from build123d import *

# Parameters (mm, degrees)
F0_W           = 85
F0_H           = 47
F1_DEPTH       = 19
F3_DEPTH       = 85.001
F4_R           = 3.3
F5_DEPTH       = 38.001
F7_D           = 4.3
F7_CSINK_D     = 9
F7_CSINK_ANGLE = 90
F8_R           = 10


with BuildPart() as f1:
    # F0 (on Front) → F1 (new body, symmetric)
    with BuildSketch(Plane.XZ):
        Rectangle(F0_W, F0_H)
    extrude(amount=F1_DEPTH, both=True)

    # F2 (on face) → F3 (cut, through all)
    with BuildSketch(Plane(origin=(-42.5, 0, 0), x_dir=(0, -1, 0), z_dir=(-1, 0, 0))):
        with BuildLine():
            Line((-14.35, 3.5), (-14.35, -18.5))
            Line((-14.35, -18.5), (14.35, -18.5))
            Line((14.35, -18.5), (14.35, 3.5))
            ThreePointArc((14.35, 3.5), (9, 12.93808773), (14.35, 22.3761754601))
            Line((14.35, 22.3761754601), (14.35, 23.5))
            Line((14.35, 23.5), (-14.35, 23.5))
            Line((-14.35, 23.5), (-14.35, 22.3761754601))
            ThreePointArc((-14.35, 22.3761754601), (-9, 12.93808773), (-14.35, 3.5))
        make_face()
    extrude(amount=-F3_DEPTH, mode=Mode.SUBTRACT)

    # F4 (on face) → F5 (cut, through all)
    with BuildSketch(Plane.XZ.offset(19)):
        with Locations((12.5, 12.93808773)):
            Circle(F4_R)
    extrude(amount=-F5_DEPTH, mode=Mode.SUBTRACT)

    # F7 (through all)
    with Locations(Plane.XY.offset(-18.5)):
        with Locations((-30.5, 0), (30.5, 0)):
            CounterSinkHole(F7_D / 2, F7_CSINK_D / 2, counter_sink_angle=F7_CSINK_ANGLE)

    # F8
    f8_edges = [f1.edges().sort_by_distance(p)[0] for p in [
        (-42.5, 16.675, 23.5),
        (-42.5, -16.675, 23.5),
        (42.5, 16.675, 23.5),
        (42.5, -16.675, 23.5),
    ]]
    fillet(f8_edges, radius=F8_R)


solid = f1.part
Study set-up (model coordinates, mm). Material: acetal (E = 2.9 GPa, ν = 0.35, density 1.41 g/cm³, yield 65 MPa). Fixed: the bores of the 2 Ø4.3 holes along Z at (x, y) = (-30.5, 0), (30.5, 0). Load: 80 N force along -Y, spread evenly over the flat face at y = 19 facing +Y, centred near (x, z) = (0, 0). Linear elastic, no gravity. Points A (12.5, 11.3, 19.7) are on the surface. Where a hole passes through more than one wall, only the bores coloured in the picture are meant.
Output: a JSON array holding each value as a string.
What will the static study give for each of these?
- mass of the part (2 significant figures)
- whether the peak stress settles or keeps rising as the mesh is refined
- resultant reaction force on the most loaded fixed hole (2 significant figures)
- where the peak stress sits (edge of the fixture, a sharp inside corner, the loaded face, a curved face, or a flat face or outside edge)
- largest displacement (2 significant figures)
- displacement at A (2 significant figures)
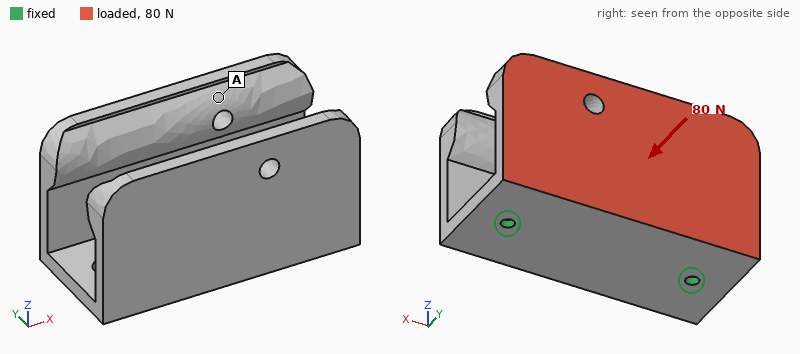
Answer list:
["85 g", "keeps rising", "40 N", "edge of the fixture", "1.1 mm", "1.0 mm"]
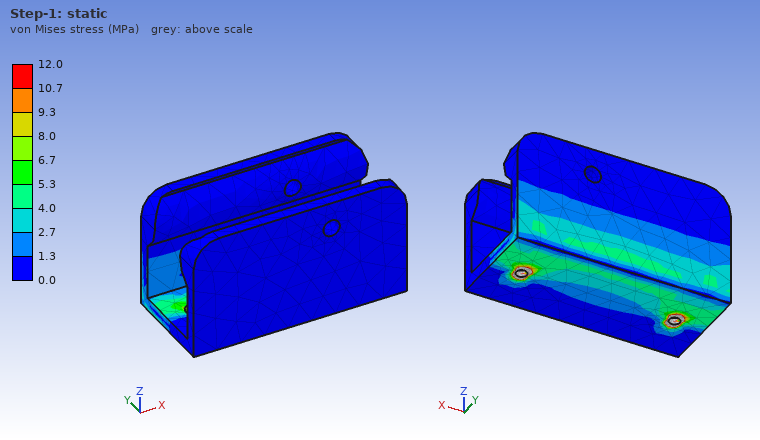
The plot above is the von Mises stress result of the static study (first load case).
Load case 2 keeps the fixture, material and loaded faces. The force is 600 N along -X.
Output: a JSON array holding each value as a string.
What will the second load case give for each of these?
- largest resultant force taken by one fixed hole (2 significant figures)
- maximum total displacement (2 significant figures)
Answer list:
["410 N", "0.73 mm"]
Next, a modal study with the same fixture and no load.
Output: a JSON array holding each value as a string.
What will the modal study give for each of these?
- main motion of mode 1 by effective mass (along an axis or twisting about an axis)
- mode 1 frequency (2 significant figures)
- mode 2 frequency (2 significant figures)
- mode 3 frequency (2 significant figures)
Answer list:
["along Y", "210 Hz", "310 Hz", "550 Hz"]
